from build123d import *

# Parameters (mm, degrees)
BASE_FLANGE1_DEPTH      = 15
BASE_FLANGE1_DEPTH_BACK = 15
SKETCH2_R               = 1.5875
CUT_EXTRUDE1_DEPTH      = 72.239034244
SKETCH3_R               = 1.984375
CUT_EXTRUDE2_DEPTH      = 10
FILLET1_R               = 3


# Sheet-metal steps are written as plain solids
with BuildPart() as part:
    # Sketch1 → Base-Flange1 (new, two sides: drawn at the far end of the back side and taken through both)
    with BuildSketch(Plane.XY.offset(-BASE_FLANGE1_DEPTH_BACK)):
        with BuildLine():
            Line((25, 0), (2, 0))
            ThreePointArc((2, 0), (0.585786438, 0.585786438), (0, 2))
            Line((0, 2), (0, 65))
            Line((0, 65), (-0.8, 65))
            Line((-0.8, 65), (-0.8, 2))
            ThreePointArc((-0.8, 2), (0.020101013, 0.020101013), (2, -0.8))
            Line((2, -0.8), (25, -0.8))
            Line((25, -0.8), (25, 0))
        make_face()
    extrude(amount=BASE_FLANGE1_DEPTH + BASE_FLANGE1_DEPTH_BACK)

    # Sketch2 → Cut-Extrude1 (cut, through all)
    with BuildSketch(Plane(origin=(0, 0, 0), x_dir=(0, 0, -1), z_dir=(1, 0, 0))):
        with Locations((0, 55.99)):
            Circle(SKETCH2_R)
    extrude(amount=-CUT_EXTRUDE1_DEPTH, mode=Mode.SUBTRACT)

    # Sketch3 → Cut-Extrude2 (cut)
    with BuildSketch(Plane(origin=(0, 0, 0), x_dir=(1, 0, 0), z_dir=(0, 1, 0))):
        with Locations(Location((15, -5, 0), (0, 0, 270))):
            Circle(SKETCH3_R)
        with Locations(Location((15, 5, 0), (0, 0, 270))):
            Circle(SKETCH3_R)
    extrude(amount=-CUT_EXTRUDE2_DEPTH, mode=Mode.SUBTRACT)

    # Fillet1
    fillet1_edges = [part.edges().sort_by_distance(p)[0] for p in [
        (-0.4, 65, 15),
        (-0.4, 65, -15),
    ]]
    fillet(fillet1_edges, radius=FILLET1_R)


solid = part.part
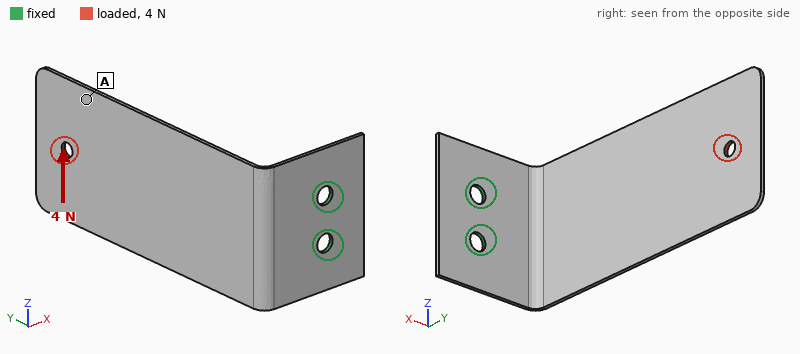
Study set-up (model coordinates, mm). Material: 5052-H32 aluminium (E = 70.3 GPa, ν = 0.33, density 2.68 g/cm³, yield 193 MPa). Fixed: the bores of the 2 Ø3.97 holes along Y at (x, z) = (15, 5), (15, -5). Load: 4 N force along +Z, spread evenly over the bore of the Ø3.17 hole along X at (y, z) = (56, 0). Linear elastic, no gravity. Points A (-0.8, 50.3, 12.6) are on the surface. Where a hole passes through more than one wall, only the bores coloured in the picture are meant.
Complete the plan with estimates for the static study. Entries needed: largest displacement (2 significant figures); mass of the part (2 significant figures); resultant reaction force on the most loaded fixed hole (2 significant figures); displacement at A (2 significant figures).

0.79 mm
5.7 g
14 N
0.61 mm
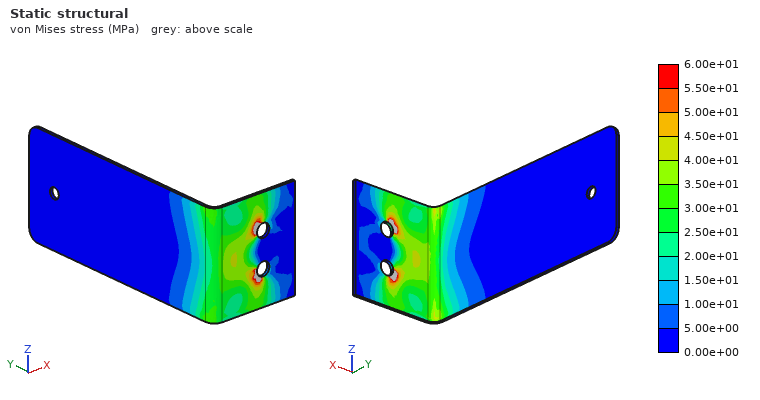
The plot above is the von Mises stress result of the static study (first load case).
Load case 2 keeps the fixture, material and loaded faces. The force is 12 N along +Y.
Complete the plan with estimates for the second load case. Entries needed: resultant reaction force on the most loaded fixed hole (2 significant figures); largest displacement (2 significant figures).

6.0 N
0.86 mm
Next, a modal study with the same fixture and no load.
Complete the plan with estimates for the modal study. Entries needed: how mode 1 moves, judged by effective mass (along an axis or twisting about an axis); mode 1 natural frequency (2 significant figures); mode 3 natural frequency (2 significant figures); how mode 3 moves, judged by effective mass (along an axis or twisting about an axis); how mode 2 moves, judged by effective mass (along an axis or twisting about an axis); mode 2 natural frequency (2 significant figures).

along X
120 Hz
710 Hz
twisting about Y
along Z
280 Hz
